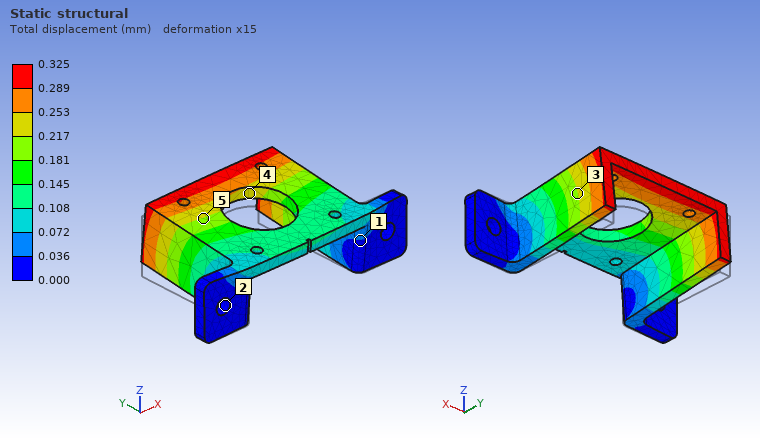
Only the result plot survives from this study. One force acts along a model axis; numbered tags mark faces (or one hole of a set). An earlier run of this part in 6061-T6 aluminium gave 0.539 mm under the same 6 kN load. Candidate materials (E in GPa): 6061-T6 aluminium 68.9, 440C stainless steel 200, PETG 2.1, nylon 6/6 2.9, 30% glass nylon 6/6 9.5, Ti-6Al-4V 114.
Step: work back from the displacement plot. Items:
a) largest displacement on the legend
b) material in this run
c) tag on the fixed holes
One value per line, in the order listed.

0.325 mm
Ti-6Al-4V
2
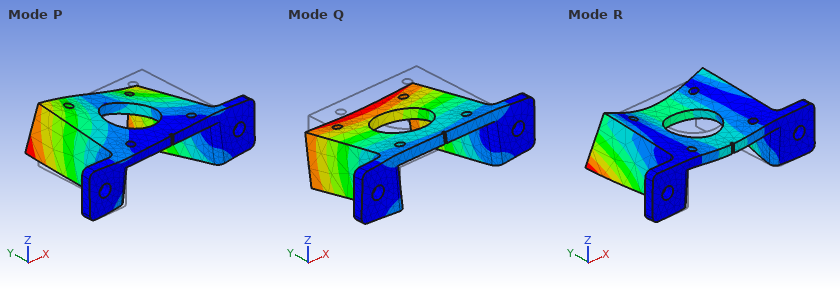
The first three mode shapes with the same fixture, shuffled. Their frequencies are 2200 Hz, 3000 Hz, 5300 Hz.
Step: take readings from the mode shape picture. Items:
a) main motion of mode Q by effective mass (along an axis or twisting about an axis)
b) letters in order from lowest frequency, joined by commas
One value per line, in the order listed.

along Z
Q, P, R
